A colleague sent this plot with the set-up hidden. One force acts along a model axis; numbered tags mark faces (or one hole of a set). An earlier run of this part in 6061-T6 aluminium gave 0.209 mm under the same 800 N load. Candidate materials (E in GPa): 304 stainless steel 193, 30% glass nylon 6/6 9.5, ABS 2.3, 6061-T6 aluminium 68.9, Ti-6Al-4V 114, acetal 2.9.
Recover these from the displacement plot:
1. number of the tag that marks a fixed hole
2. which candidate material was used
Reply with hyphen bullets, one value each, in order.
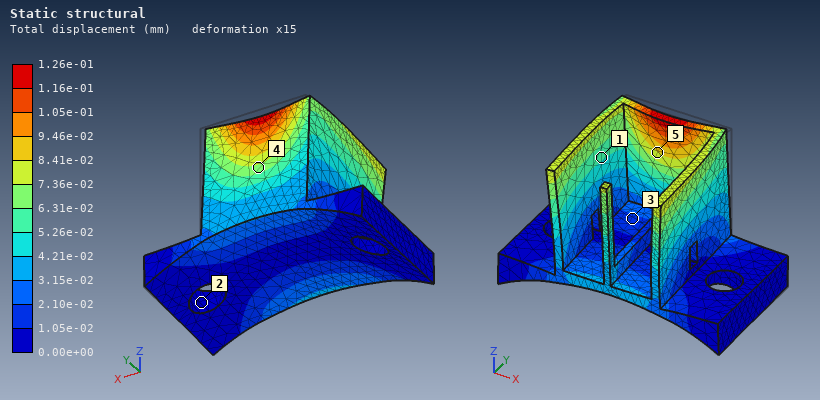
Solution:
- 2
- Ti-6Al-4V
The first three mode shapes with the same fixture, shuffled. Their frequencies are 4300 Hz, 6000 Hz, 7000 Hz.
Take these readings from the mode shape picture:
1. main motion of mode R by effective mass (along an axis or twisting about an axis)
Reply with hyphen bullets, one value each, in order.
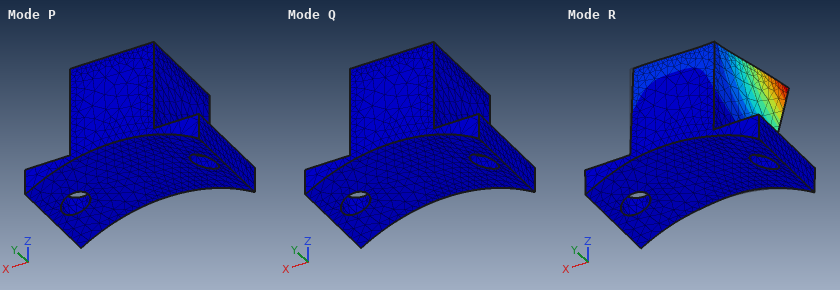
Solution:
- along X
